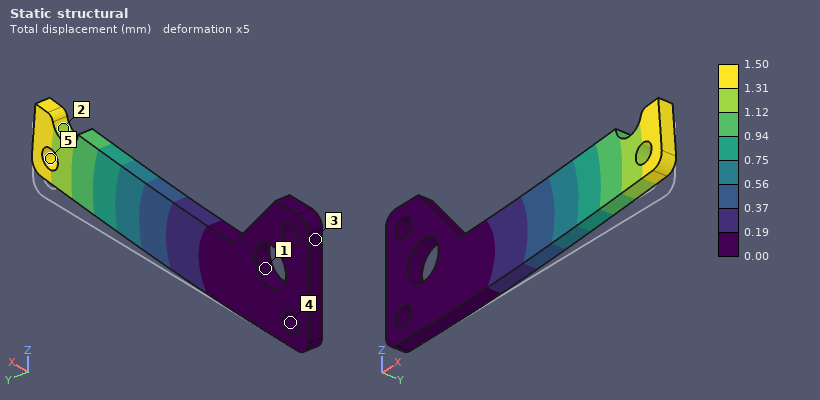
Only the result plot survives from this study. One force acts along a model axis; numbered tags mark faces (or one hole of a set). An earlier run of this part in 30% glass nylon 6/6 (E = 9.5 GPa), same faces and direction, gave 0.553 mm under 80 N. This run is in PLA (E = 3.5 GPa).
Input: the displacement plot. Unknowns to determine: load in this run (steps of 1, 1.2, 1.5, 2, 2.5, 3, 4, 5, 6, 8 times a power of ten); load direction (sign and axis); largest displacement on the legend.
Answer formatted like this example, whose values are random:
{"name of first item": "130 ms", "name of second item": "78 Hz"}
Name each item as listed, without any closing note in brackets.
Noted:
{"load in this run": "80 N", "load direction": "+Z", "largest displacement on the legend": "1.50 mm"}
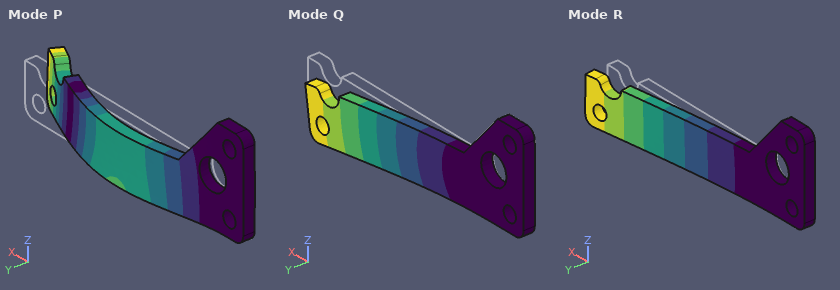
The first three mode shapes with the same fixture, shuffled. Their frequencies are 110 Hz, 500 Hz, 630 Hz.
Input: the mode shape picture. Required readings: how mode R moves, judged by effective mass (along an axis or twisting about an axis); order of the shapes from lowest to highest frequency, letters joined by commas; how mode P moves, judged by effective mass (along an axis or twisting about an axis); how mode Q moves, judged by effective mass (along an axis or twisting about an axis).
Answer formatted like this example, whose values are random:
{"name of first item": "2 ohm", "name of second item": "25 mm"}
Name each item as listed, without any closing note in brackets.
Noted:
{"how mode R moves, judged by effective mass": "along Y", "order of the shapes from lowest to highest frequency, letters joined by commas": "R, Q, P", "how mode P moves, judged by effective mass": "along Y", "how mode Q moves, judged by effective mass": "along Z"}
